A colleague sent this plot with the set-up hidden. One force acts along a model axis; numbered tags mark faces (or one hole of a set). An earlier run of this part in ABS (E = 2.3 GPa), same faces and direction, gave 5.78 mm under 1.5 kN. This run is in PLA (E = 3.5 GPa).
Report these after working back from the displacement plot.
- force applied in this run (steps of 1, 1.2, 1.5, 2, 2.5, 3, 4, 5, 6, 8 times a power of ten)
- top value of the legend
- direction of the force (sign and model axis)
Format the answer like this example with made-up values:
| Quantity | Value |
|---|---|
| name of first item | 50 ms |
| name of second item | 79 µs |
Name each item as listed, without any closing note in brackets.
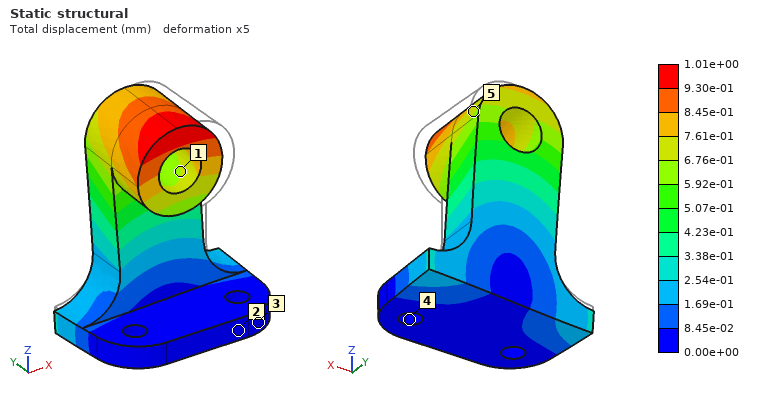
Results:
| Quantity | Value |
|---|---|
| force applied in this run | 400 N |
| top value of the legend | 1.01e+00 mm |
| direction of the force | -X |
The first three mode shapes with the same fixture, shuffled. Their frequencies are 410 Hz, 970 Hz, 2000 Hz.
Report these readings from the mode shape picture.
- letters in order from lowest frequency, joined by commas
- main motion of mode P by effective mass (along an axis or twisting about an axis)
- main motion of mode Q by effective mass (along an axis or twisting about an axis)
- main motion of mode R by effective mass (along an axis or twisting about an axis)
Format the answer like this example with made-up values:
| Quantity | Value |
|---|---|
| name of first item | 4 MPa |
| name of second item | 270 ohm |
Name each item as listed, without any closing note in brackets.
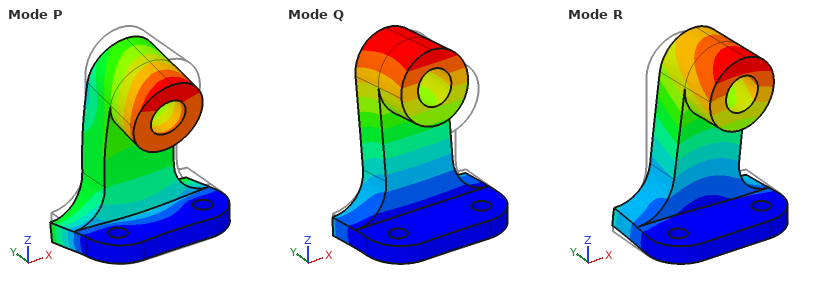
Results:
| Quantity | Value |
|---|---|
| letters in order from lowest frequency, joined by commas | Q, R, P |
| main motion of mode P by effective mass | along Z |
| main motion of mode Q by effective mass | along Y |
| main motion of mode R by effective mass | along X |
